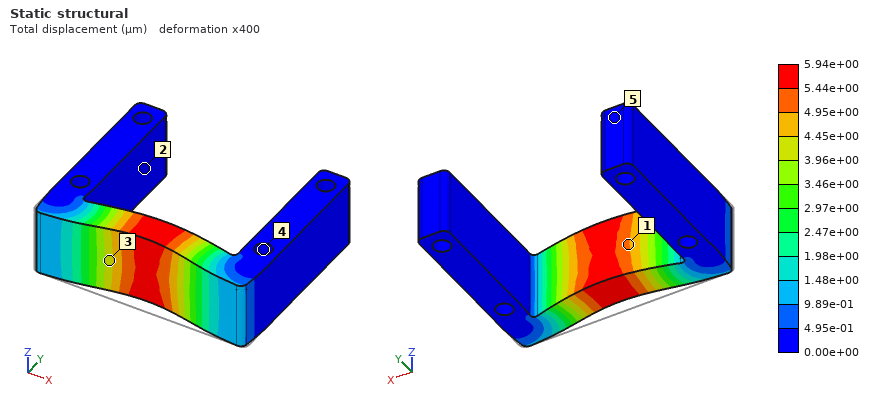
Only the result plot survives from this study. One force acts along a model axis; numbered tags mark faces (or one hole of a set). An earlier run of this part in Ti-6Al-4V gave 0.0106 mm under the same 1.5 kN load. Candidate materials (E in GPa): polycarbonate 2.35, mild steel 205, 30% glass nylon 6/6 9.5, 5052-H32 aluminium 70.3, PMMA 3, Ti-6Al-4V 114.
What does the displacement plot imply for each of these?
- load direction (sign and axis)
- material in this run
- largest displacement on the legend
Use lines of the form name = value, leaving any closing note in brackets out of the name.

load direction = +Y
material in this run = mild steel
largest displacement on the legend = 5.94e+00 µm
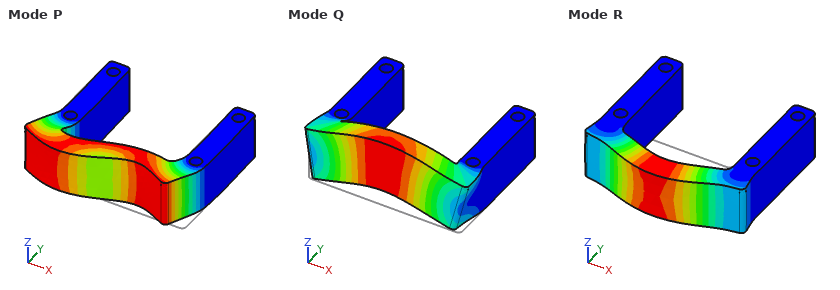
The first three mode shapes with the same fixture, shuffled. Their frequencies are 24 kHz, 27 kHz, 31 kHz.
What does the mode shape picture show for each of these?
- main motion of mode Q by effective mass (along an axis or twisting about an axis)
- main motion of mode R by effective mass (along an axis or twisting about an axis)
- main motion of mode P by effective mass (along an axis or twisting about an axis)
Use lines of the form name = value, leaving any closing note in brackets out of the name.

main motion of mode Q by effective mass = along Z
main motion of mode R by effective mass = along Y
main motion of mode P by effective mass = along X
